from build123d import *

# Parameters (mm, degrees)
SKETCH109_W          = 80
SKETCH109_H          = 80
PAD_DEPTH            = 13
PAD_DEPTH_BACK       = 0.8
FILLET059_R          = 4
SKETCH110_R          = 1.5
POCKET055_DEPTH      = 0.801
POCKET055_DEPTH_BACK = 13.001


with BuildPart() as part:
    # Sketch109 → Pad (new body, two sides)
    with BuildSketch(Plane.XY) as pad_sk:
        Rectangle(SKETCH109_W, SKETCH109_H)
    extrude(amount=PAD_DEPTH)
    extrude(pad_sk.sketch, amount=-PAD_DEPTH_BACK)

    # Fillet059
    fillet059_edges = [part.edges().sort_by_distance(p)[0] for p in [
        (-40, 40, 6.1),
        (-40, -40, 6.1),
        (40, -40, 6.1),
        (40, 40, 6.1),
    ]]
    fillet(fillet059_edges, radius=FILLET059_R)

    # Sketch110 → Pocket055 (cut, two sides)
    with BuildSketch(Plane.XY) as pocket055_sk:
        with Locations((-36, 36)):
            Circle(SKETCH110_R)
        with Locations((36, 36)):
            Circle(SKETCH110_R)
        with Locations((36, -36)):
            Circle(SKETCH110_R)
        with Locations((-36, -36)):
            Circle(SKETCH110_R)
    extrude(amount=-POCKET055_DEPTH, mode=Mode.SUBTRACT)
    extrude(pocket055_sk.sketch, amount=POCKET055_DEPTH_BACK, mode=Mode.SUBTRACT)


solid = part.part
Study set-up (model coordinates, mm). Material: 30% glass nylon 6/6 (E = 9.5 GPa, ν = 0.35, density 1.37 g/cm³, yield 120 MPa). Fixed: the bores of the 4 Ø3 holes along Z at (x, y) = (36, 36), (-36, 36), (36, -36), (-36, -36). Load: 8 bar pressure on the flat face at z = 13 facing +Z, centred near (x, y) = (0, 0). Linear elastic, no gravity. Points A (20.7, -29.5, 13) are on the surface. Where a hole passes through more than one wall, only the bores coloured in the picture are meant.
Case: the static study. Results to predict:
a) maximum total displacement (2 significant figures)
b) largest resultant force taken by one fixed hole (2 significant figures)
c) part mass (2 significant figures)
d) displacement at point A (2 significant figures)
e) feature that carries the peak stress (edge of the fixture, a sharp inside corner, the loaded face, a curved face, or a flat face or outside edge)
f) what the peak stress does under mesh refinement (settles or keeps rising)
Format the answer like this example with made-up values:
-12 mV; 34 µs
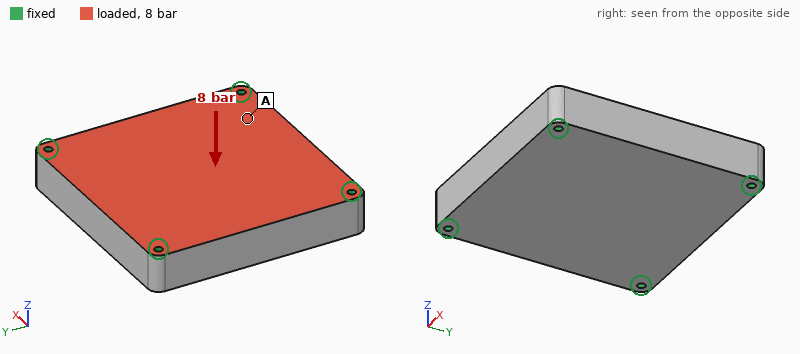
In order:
0.12 mm; 1.3 kN; 120 g; 0.064 mm; edge of the fixture; keeps rising
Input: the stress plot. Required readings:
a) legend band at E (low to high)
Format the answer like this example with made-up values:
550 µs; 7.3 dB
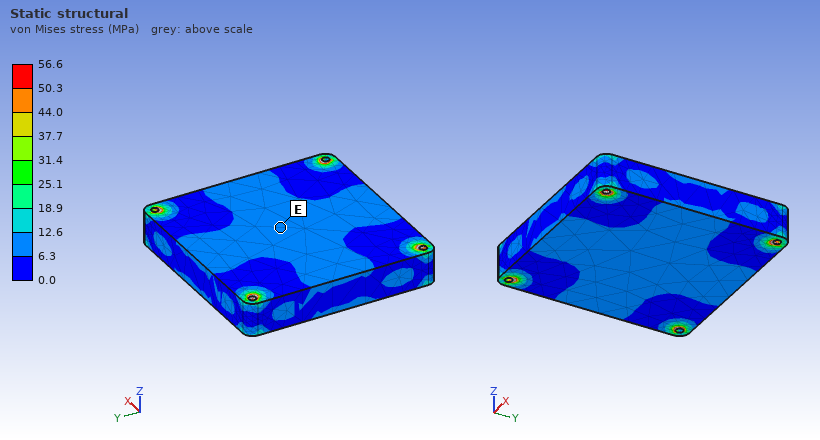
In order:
6.3 to 12.6 MPa
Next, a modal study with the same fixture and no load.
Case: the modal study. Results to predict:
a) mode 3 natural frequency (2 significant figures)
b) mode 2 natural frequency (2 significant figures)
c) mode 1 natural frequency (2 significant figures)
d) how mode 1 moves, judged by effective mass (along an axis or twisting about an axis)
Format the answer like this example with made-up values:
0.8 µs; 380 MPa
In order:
5700 Hz; 5700 Hz; 3400 Hz; along Z
